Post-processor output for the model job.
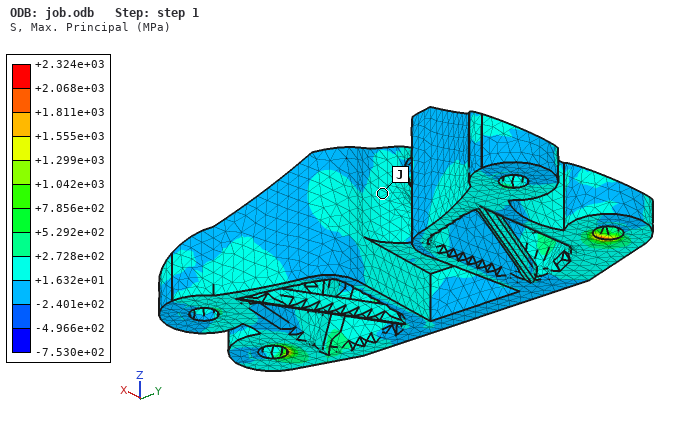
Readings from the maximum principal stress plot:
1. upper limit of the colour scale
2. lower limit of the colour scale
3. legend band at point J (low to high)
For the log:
+2.324e+03 MPa
-7.530e+02 MPa
+1.632e+01 to +2.728e+02 MPa
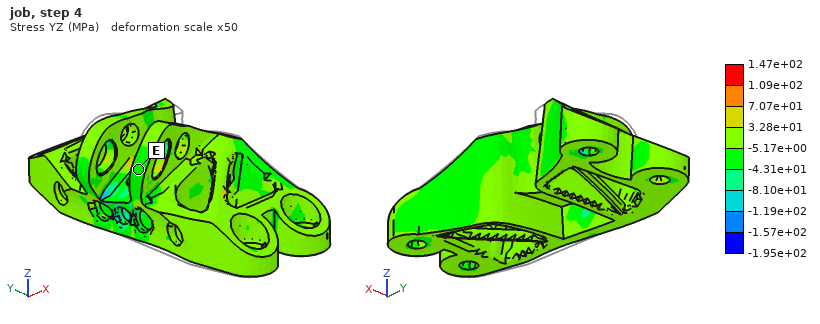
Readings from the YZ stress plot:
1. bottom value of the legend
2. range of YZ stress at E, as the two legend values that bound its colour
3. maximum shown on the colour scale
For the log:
-1.95e+02 MPa
-4.31e+01 to -5.17e+00 MPa
1.47e+02 MPa
